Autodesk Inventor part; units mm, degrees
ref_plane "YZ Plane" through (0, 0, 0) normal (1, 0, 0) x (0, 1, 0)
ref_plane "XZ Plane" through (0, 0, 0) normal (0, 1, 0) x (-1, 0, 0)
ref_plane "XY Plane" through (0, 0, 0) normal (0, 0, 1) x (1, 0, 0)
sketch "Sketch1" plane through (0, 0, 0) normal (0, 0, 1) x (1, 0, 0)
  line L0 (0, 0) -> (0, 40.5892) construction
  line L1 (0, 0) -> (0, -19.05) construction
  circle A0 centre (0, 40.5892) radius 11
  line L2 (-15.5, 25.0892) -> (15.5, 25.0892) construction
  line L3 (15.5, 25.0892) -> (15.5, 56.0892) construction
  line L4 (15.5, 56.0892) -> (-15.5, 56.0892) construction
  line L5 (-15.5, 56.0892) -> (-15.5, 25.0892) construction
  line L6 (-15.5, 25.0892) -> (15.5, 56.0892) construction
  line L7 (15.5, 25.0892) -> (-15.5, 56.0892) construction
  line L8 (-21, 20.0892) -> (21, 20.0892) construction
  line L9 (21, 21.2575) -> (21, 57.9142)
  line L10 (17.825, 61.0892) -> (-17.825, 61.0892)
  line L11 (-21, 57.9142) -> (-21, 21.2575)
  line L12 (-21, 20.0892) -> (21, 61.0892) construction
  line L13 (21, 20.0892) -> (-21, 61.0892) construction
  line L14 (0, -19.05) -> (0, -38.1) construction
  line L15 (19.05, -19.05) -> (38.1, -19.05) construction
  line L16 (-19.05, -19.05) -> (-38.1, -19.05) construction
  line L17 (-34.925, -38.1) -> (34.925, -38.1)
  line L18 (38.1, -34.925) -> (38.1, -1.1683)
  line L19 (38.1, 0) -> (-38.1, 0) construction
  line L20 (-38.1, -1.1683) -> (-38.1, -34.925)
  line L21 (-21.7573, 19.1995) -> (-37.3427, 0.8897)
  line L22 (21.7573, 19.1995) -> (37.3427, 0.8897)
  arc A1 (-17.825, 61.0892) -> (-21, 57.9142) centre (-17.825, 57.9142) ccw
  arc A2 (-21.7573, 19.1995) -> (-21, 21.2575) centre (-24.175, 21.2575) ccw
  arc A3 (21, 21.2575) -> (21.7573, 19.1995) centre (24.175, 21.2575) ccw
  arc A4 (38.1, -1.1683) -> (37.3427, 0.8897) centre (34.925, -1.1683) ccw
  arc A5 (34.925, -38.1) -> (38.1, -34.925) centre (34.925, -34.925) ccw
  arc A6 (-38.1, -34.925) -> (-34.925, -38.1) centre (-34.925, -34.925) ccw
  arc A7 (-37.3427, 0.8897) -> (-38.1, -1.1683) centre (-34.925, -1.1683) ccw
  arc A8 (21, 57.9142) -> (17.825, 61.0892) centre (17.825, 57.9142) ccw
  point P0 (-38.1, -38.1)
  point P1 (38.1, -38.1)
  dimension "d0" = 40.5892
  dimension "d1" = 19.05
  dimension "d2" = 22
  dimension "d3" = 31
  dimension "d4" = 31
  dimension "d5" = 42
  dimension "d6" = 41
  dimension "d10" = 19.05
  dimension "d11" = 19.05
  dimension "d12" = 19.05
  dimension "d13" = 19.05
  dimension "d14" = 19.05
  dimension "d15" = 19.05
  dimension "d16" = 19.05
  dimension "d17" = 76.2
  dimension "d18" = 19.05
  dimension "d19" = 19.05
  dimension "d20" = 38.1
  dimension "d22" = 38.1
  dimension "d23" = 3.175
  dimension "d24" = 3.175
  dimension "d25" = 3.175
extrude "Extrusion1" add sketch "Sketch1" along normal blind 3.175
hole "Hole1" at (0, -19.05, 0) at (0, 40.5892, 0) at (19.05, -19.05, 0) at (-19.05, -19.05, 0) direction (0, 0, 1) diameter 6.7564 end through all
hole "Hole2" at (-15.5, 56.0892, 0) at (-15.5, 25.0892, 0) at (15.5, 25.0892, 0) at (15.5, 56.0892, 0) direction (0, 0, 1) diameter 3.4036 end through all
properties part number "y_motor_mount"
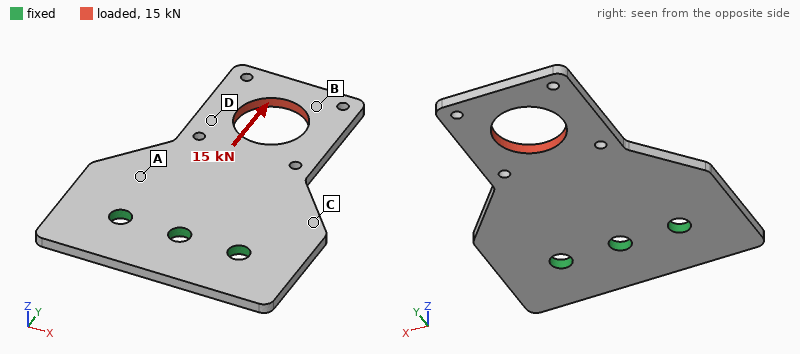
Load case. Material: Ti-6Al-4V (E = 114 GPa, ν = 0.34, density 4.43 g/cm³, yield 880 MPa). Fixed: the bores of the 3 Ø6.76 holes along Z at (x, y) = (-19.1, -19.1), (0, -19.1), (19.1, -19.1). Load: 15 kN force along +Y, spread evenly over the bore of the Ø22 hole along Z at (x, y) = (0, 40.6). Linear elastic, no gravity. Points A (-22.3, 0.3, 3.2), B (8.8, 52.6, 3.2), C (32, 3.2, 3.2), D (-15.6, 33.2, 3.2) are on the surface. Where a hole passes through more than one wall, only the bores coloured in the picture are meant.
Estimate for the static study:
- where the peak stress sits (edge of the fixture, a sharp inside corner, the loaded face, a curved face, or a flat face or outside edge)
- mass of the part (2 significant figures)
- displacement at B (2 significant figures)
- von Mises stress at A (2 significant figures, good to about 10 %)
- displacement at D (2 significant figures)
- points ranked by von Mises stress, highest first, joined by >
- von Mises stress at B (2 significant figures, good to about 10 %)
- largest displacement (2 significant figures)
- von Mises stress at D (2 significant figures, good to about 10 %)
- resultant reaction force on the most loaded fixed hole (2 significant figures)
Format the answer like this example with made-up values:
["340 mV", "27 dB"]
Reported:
["a curved face", "74 g", "0.085 mm", "72 MPa", "0.053 mm", "D > B > A > C", "98 MPa", "0.10 mm", "150 MPa", "5.5 kN"]
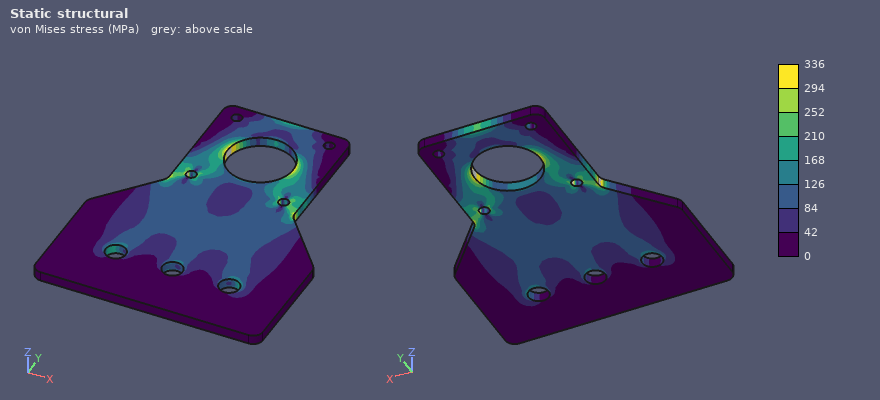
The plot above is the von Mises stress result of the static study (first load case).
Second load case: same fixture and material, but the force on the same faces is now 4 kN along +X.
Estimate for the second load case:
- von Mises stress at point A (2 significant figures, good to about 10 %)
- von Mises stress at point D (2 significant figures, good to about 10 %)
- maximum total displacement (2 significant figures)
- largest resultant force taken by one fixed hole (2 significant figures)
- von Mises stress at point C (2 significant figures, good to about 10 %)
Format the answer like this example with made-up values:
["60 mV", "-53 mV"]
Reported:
["64 MPa", "71 MPa", "0.17 mm", "5.8 kN", "34 MPa"]
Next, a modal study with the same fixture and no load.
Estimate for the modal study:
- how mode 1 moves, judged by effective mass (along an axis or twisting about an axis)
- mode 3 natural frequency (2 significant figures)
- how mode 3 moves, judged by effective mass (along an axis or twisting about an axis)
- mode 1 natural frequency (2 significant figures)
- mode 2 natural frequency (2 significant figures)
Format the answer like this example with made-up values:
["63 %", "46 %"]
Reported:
["along Z", "2500 Hz", "along Z", "580 Hz", "1800 Hz"]
